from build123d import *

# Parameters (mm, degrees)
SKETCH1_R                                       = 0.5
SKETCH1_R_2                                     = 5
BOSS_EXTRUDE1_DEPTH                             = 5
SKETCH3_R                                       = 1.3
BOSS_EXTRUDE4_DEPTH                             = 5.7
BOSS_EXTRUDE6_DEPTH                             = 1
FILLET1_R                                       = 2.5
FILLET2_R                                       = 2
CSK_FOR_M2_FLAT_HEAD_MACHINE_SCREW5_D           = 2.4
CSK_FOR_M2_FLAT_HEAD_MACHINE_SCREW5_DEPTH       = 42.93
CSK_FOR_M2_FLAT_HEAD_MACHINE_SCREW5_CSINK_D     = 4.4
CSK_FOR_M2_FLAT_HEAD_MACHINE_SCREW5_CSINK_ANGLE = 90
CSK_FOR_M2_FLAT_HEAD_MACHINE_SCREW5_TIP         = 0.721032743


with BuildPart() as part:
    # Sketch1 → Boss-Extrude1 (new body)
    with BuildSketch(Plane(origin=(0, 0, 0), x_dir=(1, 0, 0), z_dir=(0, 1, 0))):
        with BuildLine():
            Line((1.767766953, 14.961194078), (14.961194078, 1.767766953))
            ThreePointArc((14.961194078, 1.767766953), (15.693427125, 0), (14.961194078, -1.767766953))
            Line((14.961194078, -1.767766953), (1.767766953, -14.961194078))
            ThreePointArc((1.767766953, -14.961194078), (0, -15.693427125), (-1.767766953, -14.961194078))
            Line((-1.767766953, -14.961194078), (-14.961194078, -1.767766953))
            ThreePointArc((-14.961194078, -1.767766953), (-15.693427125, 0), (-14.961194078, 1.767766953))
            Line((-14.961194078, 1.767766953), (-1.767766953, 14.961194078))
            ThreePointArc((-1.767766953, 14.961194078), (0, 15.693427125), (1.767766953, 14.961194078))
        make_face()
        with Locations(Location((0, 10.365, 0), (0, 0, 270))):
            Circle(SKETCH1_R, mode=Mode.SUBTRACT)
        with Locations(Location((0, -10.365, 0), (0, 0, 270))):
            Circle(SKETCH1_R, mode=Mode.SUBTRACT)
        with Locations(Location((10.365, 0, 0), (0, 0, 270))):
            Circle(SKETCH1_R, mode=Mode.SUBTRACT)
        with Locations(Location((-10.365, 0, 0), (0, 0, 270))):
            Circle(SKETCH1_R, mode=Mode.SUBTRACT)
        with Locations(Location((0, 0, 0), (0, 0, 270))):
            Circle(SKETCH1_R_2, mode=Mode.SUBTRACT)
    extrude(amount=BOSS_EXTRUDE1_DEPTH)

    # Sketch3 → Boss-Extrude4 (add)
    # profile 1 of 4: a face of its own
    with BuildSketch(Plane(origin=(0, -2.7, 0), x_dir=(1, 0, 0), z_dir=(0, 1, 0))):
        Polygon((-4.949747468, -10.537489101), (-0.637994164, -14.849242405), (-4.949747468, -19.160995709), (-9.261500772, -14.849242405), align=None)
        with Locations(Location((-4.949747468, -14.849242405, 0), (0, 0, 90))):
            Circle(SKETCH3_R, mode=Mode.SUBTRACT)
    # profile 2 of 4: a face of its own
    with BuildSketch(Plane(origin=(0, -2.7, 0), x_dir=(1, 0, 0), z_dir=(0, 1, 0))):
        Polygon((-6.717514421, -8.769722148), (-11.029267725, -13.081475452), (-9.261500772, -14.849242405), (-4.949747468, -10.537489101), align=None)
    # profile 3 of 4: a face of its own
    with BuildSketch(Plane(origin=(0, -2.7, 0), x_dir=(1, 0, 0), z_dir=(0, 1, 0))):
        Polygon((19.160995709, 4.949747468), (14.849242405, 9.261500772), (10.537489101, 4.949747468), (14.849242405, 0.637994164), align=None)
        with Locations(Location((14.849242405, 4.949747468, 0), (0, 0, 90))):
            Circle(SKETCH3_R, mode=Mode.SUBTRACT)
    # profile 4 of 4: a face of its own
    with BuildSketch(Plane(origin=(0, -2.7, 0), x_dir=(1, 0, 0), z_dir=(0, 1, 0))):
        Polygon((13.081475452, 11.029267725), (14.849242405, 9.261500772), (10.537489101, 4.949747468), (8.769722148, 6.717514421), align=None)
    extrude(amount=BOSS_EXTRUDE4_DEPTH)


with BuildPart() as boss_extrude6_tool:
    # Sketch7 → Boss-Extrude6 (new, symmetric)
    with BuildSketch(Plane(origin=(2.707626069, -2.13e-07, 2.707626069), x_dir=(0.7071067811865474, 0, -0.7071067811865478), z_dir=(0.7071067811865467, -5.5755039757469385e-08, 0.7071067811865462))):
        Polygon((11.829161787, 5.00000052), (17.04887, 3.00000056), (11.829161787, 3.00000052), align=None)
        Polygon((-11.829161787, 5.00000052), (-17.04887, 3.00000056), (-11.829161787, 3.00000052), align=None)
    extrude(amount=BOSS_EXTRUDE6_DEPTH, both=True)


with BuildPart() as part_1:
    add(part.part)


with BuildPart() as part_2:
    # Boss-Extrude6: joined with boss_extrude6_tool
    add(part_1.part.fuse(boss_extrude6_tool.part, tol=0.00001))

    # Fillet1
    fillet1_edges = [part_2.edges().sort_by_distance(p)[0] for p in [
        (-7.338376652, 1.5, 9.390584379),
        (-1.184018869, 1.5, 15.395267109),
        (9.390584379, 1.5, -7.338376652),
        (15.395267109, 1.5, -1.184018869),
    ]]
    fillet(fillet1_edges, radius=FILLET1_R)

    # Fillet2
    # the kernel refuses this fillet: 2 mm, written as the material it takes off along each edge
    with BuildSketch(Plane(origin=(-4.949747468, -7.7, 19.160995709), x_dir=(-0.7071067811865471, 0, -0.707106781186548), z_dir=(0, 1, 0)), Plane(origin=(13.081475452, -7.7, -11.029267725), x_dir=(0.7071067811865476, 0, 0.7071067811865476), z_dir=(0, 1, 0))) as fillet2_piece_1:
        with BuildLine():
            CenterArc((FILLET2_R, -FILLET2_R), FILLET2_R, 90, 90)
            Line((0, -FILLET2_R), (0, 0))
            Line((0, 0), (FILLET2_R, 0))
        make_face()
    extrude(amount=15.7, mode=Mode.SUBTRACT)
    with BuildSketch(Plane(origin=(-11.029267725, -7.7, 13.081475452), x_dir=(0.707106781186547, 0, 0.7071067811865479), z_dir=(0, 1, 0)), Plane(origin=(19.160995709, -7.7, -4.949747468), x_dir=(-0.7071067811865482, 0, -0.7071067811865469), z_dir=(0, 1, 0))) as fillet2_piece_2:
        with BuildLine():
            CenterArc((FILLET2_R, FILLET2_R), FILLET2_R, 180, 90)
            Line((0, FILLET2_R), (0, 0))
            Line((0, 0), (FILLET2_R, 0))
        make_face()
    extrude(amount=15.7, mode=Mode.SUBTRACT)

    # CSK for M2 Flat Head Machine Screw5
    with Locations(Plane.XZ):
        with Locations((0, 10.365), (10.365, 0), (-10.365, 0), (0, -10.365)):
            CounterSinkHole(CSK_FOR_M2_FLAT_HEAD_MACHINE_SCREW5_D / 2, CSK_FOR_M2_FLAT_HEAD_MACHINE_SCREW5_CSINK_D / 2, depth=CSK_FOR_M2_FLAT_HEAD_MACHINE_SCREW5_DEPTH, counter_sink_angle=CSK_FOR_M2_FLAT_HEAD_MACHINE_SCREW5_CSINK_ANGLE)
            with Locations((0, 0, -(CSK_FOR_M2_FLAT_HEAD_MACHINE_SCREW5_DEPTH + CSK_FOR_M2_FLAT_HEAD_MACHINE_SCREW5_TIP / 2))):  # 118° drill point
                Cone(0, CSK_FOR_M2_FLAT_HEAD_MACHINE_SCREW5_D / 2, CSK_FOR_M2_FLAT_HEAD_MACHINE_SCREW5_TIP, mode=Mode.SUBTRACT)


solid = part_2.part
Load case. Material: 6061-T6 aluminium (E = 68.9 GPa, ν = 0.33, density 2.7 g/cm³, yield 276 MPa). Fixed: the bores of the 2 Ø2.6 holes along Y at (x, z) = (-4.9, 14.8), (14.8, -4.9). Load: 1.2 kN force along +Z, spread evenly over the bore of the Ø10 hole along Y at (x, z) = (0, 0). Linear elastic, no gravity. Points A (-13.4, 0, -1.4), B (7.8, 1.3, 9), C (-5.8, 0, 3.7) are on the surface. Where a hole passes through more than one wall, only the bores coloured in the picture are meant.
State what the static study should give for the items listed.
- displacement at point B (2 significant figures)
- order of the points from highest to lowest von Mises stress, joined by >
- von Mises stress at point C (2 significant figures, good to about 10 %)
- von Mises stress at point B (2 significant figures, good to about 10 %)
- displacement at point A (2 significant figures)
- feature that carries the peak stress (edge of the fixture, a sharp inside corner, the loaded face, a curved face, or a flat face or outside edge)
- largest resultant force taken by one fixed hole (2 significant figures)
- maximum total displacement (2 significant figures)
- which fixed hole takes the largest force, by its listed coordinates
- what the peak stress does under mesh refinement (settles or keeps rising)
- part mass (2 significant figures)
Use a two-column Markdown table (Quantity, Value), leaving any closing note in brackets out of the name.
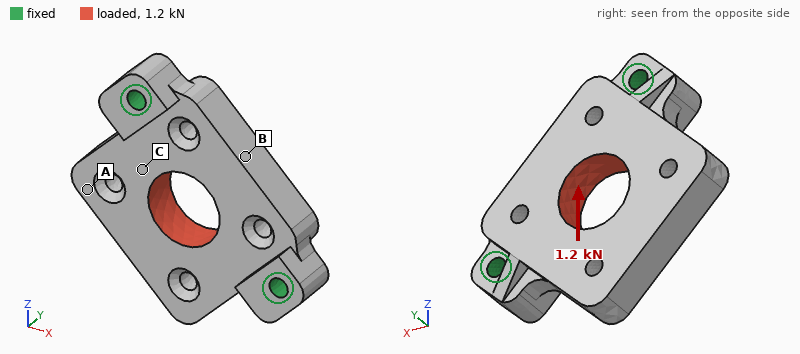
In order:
| Quantity | Value |
|---|---|
| displacement at point B | 5.5 µm |
| order of the points from highest to lowest von Mises stress, joined by > | C > B > A |
| von Mises stress at point C | 32 MPa |
| von Mises stress at point B | 15 MPa |
| displacement at point A | 11 µm |
| feature that carries the peak stress | edge of the fixture |
| largest resultant force taken by one fixed hole | 790 N |
| maximum total displacement | 12 µm |
| which fixed hole takes the largest force, by its listed coordinates | (-4.9, 14.8) |
| what the peak stress does under mesh refinement | keeps rising |
| part mass | 7.5 g |
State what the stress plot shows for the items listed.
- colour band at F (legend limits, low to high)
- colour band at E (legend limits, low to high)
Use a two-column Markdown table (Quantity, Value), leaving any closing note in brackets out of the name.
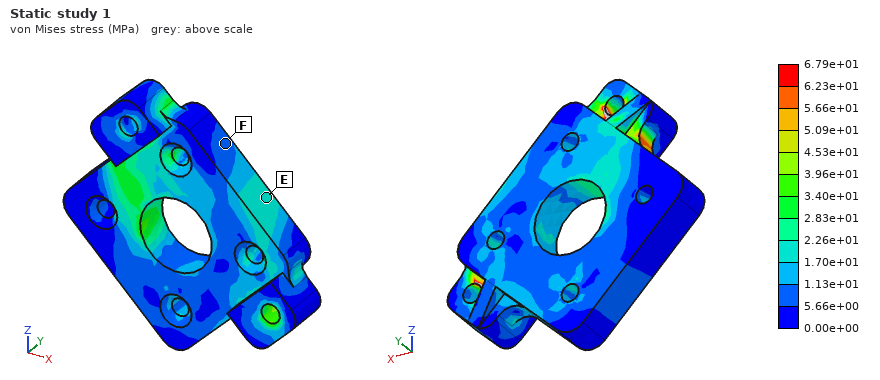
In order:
| Quantity | Value |
|---|---|
| colour band at F | 5.66e+00 to 1.13e+01 MPa |
| colour band at E | 1.70e+01 to 2.26e+01 MPa |
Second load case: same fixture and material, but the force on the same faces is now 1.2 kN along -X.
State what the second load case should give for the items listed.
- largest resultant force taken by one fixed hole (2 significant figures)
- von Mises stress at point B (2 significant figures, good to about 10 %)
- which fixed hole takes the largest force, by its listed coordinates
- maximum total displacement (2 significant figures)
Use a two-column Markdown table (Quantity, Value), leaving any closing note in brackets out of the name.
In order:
| Quantity | Value |
|---|---|
| largest resultant force taken by one fixed hole | 790 N |
| von Mises stress at point B | 19 MPa |
| which fixed hole takes the largest force, by its listed coordinates | (14.8, -4.9) |
| maximum total displacement | 12 µm |
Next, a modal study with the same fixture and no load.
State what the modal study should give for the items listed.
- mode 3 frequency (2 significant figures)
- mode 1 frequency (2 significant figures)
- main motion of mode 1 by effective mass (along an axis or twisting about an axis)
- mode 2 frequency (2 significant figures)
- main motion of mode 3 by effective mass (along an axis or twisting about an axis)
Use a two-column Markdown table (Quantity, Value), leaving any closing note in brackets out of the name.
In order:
| Quantity | Value |
|---|---|
| mode 3 frequency | 27 kHz |
| mode 1 frequency | 8300 Hz |
| main motion of mode 1 by effective mass | along Y |
| mode 2 frequency | 20 kHz |
| main motion of mode 3 by effective mass | along Y |
